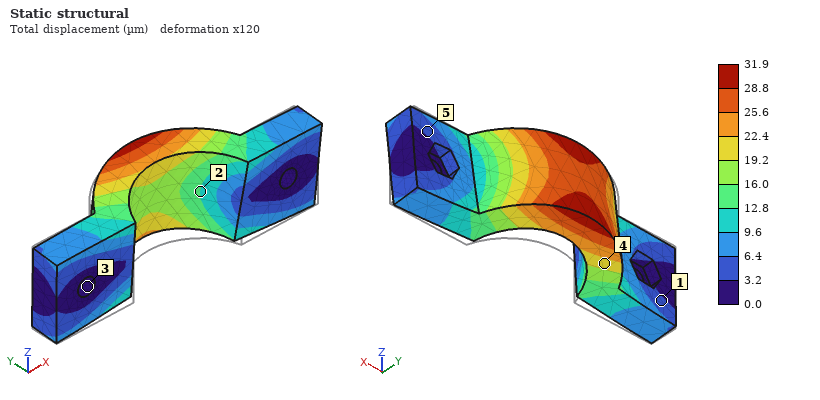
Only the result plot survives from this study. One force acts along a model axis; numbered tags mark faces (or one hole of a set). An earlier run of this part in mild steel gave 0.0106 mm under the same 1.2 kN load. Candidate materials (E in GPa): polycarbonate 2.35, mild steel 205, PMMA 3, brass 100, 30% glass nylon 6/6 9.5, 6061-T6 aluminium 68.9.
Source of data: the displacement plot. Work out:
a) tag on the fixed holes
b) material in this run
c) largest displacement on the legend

3
6061-T6 aluminium
31.9 µm
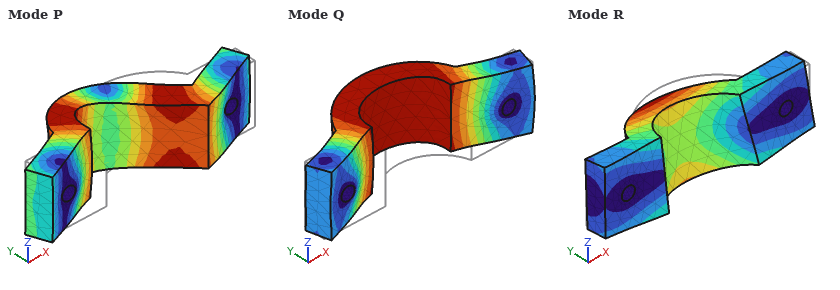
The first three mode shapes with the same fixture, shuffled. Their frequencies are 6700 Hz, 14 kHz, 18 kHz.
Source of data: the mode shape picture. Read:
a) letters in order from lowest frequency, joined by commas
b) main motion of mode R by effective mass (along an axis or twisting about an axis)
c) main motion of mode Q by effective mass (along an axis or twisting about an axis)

R, Q, P
along Z
along Y
